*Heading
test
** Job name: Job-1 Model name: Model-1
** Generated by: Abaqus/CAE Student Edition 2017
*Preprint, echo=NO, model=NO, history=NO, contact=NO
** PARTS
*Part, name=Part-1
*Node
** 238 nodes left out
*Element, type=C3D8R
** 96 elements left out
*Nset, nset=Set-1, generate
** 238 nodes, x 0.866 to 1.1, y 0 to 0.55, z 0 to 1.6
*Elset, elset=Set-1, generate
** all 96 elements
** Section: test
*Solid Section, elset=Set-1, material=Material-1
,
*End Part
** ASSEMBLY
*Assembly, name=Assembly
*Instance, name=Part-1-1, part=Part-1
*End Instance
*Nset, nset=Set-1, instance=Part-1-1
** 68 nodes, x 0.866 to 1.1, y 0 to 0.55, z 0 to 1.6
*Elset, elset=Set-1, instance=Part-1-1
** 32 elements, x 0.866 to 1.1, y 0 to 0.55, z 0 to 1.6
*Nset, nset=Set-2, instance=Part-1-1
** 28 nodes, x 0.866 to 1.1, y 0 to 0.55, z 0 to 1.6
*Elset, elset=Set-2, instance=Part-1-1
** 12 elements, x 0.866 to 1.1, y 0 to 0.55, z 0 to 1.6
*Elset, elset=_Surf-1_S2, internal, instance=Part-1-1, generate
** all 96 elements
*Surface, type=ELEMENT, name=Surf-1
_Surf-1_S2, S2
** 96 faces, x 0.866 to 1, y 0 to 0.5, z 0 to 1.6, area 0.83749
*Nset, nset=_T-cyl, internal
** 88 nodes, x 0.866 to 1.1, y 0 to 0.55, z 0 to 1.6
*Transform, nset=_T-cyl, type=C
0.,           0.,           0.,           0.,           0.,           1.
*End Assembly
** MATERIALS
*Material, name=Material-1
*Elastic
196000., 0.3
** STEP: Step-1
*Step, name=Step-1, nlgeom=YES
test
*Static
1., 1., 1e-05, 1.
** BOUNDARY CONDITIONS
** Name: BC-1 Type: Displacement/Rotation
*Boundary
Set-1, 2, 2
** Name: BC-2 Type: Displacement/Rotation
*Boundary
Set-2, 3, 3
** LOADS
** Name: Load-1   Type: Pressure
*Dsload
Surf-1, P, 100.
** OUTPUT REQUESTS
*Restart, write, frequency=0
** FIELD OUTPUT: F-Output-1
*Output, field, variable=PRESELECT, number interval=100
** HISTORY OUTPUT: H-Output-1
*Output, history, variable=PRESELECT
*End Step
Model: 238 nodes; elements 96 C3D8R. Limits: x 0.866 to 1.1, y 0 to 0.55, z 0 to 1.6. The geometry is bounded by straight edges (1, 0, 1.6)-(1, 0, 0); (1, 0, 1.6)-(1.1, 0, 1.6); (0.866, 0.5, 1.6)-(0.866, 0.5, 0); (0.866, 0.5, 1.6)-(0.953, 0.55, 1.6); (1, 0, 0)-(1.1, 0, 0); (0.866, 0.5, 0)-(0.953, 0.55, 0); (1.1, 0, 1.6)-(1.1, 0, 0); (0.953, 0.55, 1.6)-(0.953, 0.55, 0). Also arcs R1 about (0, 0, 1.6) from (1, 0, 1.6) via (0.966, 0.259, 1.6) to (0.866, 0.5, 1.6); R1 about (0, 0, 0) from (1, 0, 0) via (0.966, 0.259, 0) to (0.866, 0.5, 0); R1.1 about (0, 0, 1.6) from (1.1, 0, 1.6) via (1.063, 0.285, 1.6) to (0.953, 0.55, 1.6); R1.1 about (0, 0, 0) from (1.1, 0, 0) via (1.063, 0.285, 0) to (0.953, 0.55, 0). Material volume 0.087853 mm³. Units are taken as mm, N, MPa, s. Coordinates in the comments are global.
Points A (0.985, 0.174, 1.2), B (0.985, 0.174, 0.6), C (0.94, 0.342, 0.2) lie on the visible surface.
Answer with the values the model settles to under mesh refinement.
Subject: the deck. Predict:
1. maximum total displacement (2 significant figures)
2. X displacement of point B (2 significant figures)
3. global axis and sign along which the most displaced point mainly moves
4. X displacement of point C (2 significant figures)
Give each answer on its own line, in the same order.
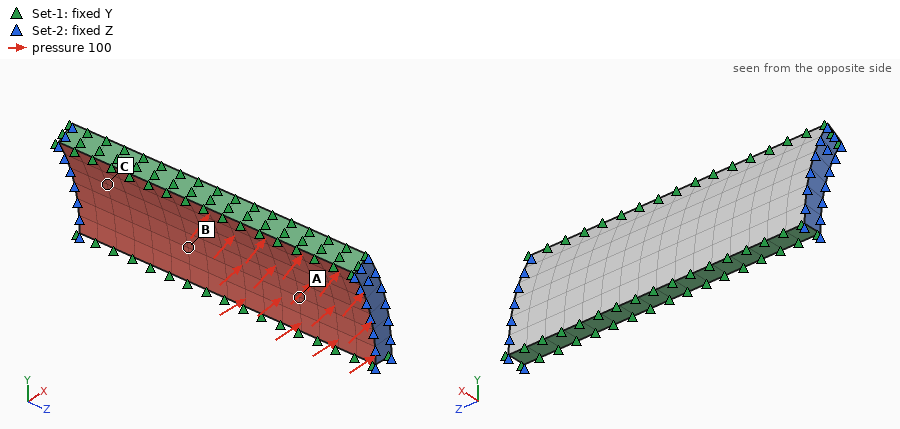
0.0051 mm
0.0050 mm
+X
0.0048 mm
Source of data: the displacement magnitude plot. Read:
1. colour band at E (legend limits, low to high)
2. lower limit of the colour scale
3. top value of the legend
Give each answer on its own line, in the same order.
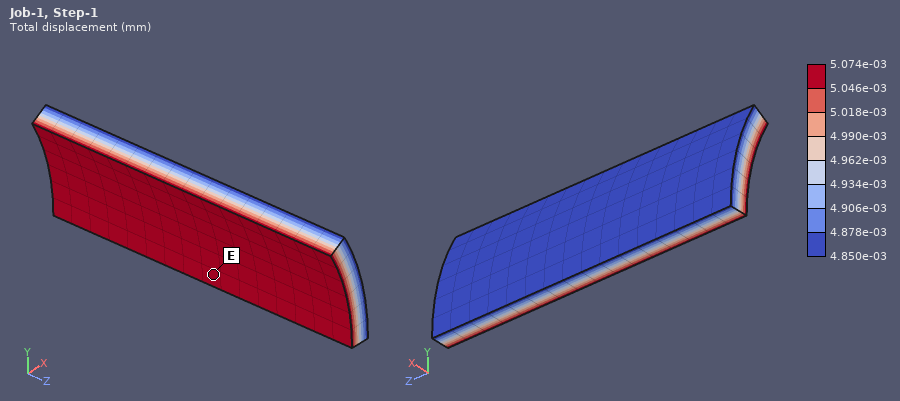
5.046e-03 to 5.074e-03 mm
4.850e-03 mm
5.074e-03 mm
